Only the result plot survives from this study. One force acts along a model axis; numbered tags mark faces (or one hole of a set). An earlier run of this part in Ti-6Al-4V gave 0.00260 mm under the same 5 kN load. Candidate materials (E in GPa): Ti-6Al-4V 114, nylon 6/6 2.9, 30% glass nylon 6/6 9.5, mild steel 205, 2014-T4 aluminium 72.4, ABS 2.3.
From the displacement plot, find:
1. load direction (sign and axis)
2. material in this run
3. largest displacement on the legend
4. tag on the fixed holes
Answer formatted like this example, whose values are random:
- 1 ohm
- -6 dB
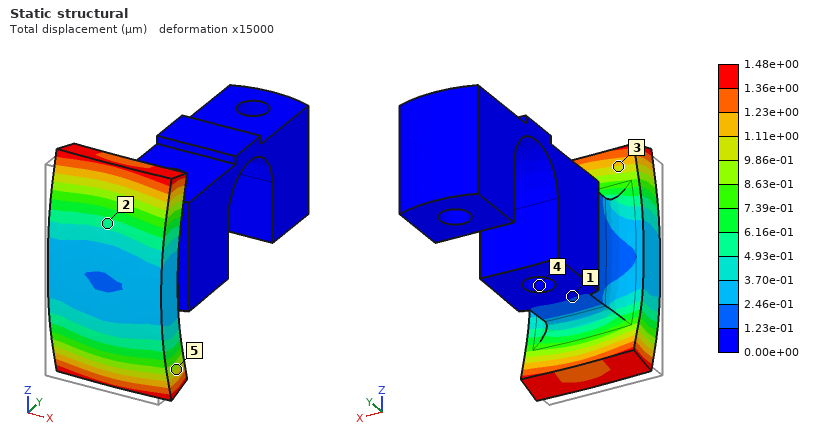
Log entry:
- +Y
- mild steel
- 1.48e+00 µm
- 4
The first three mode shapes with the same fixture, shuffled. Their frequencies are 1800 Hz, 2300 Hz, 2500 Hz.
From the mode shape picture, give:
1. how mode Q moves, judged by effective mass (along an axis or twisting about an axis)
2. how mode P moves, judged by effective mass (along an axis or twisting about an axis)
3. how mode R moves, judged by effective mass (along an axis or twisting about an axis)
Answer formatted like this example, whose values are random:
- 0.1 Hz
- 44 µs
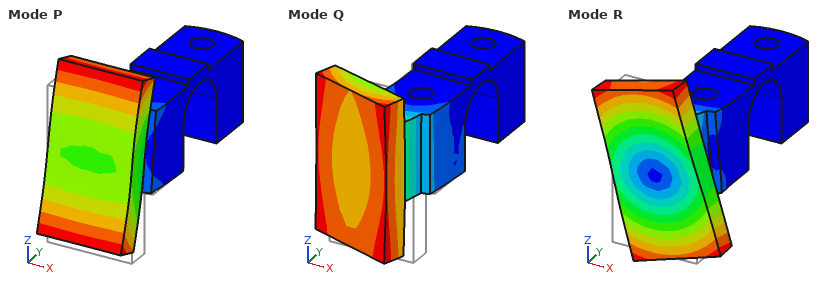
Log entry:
- along X
- along Z
- twisting about Y
